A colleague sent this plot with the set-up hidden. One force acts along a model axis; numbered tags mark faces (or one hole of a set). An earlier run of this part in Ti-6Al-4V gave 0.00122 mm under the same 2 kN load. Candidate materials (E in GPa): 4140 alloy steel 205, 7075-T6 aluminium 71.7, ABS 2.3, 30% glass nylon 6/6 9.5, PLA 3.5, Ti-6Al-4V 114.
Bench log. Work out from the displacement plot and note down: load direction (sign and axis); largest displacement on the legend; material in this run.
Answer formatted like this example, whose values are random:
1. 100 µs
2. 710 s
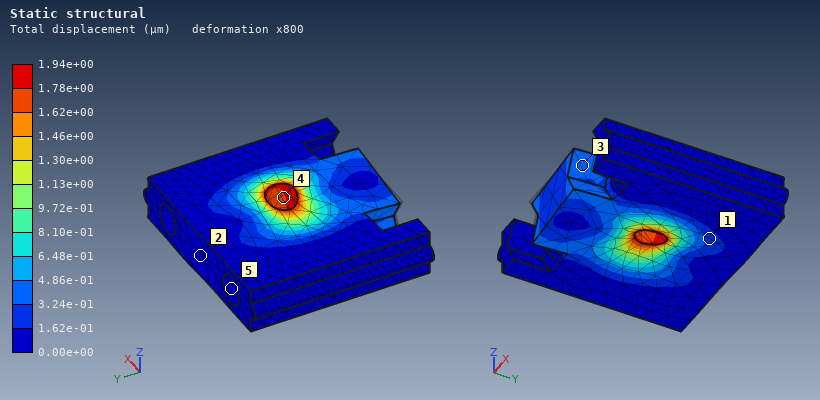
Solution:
1. +X
2. 1.94e+00 µm
3. 7075-T6 aluminium
